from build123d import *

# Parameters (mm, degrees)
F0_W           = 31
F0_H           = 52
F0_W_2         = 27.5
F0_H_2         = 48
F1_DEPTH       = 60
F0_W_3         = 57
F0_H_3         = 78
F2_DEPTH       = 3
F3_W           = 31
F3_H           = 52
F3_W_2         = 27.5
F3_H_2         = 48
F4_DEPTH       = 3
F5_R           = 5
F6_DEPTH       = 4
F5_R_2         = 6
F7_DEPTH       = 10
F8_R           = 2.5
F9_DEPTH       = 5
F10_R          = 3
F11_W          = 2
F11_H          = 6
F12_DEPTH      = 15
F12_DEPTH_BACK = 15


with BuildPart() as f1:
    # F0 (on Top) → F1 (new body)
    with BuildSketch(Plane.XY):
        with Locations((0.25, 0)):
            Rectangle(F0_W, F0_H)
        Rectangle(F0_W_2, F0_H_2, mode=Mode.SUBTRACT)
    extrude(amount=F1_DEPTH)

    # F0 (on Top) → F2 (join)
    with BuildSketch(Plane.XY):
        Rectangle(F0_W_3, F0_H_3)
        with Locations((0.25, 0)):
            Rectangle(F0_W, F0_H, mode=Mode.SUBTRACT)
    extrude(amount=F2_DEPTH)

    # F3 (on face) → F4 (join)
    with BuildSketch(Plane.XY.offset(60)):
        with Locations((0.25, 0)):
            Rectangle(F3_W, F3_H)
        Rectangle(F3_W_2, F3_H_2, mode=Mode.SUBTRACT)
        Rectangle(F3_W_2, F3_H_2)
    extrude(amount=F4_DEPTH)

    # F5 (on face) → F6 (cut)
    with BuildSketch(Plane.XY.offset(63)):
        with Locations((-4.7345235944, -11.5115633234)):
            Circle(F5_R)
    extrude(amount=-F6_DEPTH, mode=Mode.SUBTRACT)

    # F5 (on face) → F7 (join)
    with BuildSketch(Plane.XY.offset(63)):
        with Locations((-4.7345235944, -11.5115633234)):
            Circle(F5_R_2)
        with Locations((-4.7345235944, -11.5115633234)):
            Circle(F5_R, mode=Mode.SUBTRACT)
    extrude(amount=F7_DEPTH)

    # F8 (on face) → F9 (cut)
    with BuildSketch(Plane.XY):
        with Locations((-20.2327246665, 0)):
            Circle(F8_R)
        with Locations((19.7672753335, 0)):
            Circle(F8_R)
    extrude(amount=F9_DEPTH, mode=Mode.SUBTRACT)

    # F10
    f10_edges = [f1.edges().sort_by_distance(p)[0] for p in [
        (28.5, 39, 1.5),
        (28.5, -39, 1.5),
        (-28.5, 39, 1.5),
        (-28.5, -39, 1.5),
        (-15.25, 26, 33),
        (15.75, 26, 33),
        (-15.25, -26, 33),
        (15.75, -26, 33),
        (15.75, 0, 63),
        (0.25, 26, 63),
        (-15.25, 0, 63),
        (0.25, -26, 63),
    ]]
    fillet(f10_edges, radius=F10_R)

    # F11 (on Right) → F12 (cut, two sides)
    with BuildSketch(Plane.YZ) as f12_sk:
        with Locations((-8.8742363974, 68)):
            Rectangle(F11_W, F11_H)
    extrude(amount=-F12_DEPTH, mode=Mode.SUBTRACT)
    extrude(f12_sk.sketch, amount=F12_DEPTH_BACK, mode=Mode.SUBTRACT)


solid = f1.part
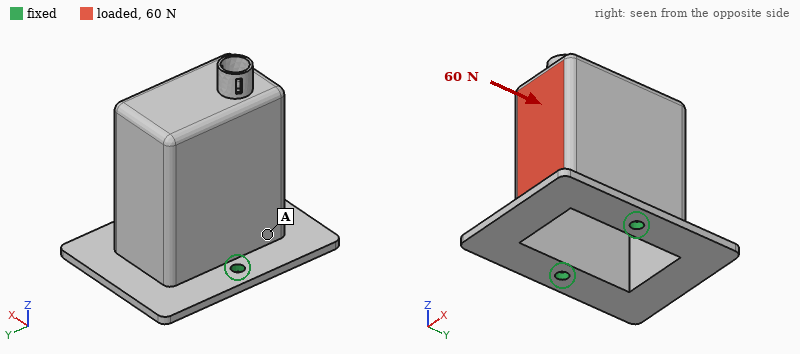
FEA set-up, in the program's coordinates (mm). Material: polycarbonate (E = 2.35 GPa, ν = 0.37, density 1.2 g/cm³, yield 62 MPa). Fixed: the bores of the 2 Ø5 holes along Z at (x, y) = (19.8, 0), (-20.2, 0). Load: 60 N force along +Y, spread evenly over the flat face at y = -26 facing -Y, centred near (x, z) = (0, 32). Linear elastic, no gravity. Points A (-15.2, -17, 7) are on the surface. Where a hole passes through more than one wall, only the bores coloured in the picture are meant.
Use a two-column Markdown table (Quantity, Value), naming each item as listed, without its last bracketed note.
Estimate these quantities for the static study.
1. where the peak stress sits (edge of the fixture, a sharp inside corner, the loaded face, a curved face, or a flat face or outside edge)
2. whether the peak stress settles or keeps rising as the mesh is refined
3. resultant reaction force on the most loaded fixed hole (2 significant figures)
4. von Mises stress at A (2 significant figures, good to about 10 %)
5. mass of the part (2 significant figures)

| Quantity | Value |
|---|---|
| where the peak stress sits | edge of the fixture |
| whether the peak stress settles or keeps rising as the mesh is refined | keeps rising |
| resultant reaction force on the most loaded fixed hole | 32 N |
| von Mises stress at A | 1.9 MPa |
| mass of the part | 36 g |
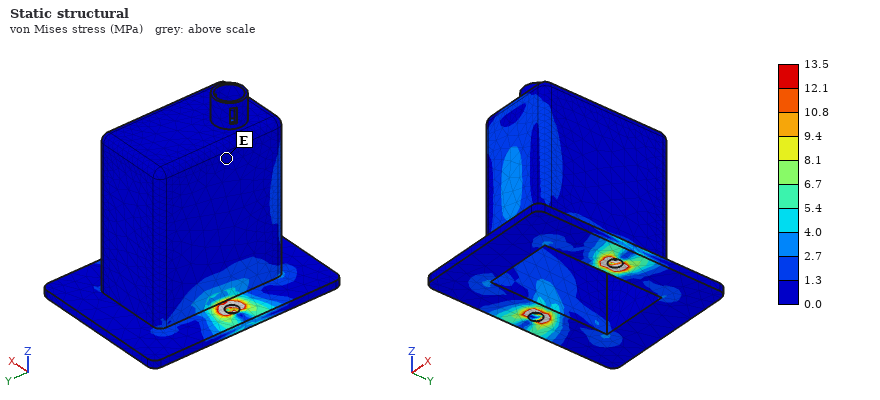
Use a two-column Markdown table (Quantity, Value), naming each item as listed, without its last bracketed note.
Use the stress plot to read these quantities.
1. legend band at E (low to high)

| Quantity | Value |
|---|---|
| legend band at E | 0.0 to 1.3 MPa |
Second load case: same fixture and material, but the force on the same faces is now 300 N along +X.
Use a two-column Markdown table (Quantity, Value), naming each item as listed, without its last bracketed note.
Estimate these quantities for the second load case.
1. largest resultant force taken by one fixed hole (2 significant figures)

| Quantity | Value |
|---|---|
| largest resultant force taken by one fixed hole | 340 N |
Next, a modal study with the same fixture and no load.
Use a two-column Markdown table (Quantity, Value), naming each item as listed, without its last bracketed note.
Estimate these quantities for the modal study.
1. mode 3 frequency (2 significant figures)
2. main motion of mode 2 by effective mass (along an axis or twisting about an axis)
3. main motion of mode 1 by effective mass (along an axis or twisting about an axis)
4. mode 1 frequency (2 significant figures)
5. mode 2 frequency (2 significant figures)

| Quantity | Value |
|---|---|
| mode 3 frequency | 1100 Hz |
| main motion of mode 2 by effective mass | along X |
| main motion of mode 1 by effective mass | along Y |
| mode 1 frequency | 210 Hz |
| mode 2 frequency | 580 Hz |
